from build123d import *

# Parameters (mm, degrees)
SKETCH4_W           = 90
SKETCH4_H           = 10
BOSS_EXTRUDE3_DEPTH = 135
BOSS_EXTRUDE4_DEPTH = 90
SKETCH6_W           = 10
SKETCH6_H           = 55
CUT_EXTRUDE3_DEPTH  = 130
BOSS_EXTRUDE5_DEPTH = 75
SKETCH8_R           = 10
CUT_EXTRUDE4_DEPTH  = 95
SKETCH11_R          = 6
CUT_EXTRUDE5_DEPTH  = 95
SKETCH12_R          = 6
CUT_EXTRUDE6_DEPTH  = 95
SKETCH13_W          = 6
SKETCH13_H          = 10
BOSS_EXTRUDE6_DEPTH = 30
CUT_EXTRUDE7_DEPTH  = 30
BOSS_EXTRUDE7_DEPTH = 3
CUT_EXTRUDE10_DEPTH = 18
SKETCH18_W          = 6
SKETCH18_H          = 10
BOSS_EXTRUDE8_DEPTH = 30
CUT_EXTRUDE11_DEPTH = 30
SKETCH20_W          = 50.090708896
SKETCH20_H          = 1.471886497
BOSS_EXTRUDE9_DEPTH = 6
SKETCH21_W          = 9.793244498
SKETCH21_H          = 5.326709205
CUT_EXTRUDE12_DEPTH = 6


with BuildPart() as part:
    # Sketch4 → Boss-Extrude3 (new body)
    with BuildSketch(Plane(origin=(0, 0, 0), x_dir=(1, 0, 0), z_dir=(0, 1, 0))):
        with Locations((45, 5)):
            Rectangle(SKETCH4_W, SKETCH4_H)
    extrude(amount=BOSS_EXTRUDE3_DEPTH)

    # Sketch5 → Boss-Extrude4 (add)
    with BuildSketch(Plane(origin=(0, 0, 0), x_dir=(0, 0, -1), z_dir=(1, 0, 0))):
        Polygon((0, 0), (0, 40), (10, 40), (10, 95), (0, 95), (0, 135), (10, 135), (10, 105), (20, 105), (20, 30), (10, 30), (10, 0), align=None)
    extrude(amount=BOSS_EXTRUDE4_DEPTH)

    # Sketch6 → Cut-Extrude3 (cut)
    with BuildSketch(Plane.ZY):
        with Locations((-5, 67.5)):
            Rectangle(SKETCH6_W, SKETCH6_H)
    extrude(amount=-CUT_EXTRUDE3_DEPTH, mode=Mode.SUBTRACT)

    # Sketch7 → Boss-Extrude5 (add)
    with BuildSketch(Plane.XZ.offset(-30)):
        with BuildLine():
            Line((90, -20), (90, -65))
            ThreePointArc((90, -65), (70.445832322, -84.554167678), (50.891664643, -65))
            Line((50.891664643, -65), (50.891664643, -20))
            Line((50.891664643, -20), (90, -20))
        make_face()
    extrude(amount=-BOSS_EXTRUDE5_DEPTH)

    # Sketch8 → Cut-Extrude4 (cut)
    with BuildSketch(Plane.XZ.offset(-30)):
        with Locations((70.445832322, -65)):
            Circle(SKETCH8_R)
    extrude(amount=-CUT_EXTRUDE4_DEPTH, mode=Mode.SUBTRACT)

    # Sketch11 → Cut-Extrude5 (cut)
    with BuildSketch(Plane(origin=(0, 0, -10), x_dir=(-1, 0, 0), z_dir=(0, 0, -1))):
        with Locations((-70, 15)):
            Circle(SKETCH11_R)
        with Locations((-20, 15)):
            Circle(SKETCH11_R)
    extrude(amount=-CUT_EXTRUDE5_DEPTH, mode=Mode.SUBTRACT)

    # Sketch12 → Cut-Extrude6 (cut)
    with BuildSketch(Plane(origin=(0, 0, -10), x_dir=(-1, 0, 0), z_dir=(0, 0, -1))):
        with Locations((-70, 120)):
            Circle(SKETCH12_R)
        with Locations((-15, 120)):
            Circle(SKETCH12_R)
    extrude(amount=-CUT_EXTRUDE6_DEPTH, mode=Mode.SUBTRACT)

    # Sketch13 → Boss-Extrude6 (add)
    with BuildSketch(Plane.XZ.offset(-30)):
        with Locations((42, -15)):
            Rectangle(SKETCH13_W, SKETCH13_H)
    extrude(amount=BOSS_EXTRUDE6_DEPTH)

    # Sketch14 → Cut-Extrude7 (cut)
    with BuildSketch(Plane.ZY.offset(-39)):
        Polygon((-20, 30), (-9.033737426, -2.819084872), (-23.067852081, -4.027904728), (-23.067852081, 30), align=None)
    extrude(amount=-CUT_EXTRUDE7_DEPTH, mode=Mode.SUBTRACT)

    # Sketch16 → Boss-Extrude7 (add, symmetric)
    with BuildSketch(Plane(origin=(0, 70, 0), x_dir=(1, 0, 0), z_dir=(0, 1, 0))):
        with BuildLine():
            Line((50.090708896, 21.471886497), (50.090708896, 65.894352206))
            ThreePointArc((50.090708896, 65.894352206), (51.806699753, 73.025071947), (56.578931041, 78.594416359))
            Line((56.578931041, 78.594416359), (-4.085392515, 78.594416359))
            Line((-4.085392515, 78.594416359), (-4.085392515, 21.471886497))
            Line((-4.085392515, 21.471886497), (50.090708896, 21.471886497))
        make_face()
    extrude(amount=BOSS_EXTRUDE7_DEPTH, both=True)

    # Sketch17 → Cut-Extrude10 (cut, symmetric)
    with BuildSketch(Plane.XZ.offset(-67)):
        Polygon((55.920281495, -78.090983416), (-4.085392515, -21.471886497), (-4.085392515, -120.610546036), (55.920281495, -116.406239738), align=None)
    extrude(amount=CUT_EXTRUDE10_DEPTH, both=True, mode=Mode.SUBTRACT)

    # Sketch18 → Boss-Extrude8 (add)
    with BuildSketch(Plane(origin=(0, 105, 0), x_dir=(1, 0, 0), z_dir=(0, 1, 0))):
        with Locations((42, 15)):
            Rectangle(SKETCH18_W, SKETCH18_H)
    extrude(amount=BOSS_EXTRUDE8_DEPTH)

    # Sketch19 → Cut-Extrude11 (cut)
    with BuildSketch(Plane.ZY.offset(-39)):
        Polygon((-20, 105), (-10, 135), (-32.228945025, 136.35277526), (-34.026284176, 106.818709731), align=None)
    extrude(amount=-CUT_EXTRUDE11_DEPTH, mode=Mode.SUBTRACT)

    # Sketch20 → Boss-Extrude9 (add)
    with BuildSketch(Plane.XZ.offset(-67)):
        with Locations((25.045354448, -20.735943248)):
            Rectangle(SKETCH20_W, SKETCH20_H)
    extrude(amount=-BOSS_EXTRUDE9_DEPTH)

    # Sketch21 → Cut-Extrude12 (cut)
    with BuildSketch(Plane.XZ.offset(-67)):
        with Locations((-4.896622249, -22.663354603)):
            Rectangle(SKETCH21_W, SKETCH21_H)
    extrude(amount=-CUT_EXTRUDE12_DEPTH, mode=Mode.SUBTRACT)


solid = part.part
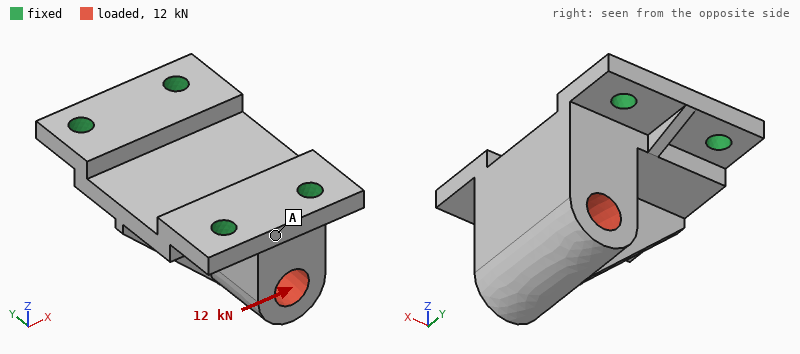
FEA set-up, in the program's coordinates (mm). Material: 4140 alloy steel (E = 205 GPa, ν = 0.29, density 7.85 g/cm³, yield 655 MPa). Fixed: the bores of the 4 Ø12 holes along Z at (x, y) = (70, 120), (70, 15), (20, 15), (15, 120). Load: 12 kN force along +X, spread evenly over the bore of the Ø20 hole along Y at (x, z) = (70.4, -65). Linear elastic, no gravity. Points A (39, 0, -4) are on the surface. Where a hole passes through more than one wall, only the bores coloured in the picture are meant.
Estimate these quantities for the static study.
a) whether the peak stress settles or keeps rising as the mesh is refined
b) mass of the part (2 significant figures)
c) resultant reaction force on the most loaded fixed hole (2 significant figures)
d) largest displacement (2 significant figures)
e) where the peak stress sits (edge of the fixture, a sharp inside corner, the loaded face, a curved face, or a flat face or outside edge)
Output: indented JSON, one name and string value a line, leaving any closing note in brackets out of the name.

{
  "whether the peak stress settles or keeps rising as the mesh is refined": "keeps rising",
  "mass of the part": "2.3 kg",
  "resultant reaction force on the most loaded fixed hole": "11 kN",
  "largest displacement": "0.10 mm",
  "where the peak stress sits": "edge of the fixture"
}
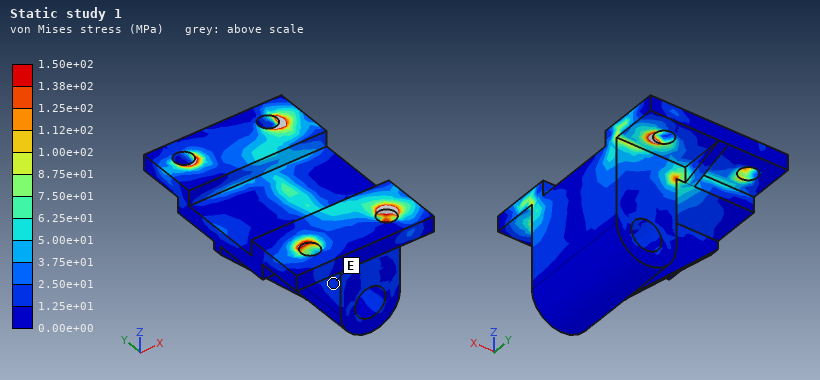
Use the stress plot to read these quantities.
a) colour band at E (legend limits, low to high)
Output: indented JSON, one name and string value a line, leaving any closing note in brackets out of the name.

{
  "colour band at E": "1.25e+01 to 2.50e+01 MPa"
}
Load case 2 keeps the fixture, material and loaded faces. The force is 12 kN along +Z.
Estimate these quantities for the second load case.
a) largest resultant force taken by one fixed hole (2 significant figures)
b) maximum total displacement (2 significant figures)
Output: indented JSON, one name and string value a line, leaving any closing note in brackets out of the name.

{
  "largest resultant force taken by one fixed hole": "7.1 kN",
  "maximum total displacement": "18 µm"
}
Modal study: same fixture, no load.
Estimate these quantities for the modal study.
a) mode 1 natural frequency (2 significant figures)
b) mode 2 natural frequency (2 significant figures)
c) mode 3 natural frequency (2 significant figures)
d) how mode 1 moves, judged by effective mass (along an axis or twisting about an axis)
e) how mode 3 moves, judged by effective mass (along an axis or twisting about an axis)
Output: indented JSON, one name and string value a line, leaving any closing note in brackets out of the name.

{
  "mode 1 natural frequency": "2300 Hz",
  "mode 2 natural frequency": "2900 Hz",
  "mode 3 natural frequency": "4200 Hz",
  "how mode 1 moves, judged by effective mass": "along X",
  "how mode 3 moves, judged by effective mass": "along Y"
}
